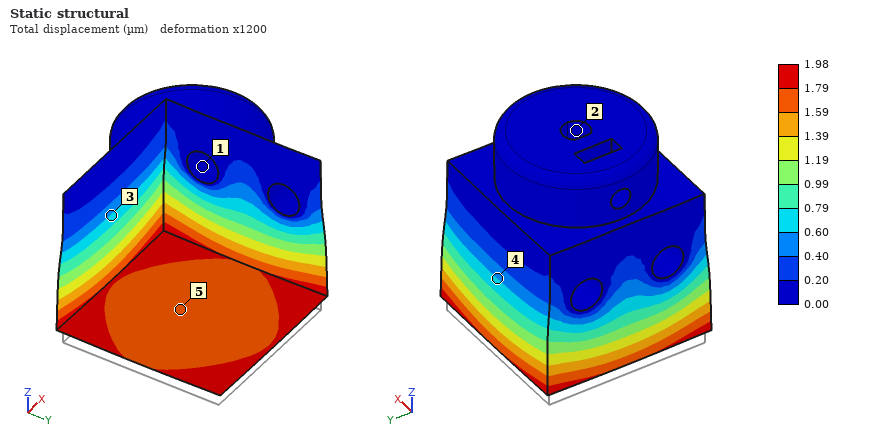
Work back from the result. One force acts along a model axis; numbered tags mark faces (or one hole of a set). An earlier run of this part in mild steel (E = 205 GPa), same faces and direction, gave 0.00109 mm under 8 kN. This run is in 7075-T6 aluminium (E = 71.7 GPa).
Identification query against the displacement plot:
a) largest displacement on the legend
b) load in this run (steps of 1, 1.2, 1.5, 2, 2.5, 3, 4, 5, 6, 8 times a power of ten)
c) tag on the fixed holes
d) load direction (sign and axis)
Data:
1.98 µm
5 kN
1
+Z
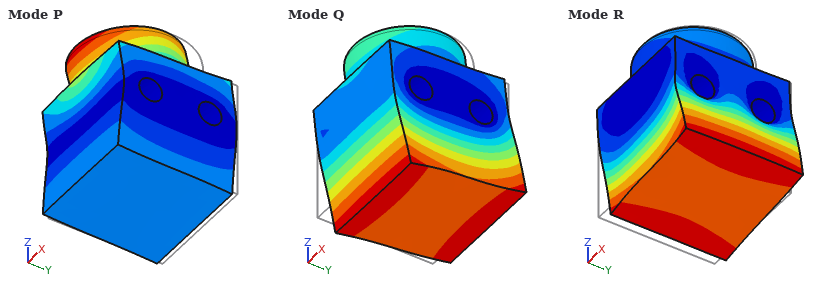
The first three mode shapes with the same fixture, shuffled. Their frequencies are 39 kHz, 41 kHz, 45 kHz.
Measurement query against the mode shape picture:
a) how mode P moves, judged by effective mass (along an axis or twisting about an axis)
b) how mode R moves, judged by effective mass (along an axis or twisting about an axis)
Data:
along Y
along X
